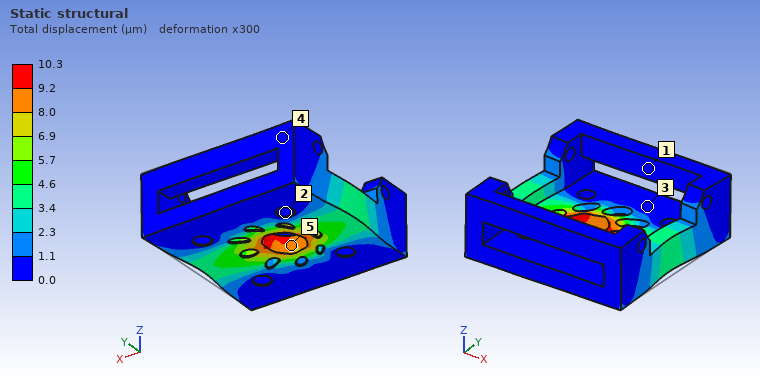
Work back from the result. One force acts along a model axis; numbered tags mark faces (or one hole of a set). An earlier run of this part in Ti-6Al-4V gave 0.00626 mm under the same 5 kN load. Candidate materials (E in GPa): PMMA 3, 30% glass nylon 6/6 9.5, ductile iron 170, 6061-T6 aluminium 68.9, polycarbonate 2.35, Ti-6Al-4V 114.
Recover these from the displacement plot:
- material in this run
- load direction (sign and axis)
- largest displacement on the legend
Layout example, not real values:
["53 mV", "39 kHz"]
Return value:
["6061-T6 aluminium", "-X", "10.3 µm"]
